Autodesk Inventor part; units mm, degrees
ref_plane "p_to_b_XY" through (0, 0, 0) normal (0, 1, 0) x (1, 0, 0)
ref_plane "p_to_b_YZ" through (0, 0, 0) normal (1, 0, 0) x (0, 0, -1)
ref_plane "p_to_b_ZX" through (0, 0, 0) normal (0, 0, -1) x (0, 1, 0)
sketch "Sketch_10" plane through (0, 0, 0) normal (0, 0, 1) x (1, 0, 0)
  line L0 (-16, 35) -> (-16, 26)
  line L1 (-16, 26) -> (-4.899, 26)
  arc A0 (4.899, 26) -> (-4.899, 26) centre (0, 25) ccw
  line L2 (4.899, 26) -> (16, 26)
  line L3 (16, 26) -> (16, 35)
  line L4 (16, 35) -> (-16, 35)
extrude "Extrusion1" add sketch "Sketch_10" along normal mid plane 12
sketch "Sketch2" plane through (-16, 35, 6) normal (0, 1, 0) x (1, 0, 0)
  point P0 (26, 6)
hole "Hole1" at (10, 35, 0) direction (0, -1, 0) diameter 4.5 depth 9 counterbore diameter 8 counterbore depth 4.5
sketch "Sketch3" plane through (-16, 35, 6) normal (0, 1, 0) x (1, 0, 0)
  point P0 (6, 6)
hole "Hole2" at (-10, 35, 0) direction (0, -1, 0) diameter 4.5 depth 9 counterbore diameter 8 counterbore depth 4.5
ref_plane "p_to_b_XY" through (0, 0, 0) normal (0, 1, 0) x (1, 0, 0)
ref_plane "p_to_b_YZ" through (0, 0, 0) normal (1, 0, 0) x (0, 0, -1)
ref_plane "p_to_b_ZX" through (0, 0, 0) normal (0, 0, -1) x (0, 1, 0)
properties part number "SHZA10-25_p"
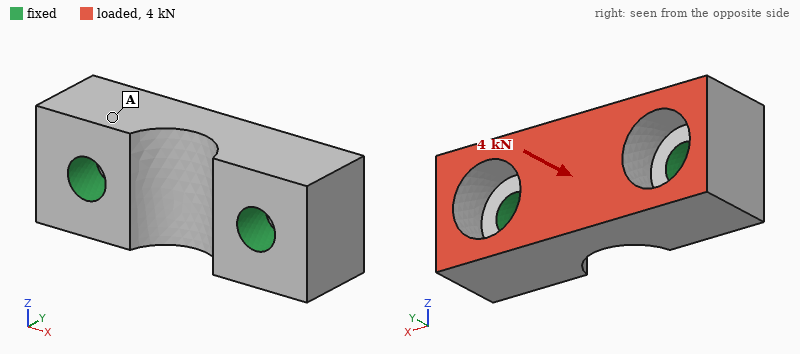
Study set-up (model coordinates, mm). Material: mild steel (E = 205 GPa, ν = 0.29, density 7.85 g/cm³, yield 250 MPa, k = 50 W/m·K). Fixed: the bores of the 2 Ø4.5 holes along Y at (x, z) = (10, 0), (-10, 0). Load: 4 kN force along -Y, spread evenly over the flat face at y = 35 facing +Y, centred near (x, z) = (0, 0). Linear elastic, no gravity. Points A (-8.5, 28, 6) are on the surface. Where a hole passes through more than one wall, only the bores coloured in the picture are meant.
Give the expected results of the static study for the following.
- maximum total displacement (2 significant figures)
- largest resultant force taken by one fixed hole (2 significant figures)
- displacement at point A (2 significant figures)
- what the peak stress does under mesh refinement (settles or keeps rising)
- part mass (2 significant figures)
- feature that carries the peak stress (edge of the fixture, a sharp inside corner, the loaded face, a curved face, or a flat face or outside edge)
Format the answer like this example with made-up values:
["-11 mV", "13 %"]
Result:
["2.6 µm", "2.1 kN", "1.2 µm", "keeps rising", "20 g", "edge of the fixture"]
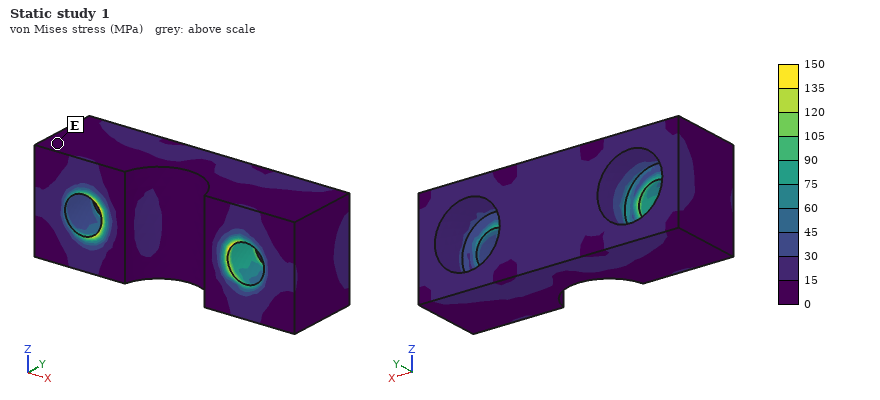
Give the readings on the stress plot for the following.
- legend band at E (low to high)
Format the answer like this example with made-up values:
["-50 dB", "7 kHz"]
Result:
["0 to 15 MPa"]
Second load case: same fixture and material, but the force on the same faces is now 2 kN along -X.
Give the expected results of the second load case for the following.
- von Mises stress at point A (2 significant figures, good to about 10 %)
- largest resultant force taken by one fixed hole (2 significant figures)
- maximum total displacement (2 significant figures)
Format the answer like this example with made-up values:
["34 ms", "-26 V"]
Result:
["9.3 MPa", "1.1 kN", "2.7 µm"]
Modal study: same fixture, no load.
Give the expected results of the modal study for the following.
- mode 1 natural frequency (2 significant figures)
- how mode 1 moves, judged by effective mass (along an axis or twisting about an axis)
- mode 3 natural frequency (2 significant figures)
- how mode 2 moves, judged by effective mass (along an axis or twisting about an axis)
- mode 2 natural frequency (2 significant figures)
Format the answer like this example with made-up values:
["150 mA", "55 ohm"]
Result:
["37 kHz", "along Z", "55 kHz", "twisting about Y", "53 kHz"]
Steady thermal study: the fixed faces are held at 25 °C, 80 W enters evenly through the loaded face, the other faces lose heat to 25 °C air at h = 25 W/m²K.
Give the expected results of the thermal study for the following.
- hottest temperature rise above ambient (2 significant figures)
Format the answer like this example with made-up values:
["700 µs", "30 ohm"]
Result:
["75 K"]
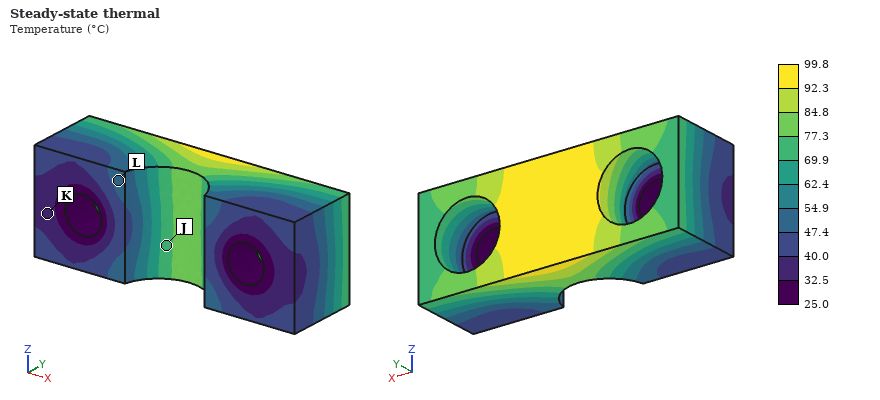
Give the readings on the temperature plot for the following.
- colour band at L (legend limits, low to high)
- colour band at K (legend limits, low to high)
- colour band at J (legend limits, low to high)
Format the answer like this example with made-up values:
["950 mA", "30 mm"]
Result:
["47.4 to 54.9 °C", "32.5 to 40.0 °C", "69.9 to 77.3 °C"]
